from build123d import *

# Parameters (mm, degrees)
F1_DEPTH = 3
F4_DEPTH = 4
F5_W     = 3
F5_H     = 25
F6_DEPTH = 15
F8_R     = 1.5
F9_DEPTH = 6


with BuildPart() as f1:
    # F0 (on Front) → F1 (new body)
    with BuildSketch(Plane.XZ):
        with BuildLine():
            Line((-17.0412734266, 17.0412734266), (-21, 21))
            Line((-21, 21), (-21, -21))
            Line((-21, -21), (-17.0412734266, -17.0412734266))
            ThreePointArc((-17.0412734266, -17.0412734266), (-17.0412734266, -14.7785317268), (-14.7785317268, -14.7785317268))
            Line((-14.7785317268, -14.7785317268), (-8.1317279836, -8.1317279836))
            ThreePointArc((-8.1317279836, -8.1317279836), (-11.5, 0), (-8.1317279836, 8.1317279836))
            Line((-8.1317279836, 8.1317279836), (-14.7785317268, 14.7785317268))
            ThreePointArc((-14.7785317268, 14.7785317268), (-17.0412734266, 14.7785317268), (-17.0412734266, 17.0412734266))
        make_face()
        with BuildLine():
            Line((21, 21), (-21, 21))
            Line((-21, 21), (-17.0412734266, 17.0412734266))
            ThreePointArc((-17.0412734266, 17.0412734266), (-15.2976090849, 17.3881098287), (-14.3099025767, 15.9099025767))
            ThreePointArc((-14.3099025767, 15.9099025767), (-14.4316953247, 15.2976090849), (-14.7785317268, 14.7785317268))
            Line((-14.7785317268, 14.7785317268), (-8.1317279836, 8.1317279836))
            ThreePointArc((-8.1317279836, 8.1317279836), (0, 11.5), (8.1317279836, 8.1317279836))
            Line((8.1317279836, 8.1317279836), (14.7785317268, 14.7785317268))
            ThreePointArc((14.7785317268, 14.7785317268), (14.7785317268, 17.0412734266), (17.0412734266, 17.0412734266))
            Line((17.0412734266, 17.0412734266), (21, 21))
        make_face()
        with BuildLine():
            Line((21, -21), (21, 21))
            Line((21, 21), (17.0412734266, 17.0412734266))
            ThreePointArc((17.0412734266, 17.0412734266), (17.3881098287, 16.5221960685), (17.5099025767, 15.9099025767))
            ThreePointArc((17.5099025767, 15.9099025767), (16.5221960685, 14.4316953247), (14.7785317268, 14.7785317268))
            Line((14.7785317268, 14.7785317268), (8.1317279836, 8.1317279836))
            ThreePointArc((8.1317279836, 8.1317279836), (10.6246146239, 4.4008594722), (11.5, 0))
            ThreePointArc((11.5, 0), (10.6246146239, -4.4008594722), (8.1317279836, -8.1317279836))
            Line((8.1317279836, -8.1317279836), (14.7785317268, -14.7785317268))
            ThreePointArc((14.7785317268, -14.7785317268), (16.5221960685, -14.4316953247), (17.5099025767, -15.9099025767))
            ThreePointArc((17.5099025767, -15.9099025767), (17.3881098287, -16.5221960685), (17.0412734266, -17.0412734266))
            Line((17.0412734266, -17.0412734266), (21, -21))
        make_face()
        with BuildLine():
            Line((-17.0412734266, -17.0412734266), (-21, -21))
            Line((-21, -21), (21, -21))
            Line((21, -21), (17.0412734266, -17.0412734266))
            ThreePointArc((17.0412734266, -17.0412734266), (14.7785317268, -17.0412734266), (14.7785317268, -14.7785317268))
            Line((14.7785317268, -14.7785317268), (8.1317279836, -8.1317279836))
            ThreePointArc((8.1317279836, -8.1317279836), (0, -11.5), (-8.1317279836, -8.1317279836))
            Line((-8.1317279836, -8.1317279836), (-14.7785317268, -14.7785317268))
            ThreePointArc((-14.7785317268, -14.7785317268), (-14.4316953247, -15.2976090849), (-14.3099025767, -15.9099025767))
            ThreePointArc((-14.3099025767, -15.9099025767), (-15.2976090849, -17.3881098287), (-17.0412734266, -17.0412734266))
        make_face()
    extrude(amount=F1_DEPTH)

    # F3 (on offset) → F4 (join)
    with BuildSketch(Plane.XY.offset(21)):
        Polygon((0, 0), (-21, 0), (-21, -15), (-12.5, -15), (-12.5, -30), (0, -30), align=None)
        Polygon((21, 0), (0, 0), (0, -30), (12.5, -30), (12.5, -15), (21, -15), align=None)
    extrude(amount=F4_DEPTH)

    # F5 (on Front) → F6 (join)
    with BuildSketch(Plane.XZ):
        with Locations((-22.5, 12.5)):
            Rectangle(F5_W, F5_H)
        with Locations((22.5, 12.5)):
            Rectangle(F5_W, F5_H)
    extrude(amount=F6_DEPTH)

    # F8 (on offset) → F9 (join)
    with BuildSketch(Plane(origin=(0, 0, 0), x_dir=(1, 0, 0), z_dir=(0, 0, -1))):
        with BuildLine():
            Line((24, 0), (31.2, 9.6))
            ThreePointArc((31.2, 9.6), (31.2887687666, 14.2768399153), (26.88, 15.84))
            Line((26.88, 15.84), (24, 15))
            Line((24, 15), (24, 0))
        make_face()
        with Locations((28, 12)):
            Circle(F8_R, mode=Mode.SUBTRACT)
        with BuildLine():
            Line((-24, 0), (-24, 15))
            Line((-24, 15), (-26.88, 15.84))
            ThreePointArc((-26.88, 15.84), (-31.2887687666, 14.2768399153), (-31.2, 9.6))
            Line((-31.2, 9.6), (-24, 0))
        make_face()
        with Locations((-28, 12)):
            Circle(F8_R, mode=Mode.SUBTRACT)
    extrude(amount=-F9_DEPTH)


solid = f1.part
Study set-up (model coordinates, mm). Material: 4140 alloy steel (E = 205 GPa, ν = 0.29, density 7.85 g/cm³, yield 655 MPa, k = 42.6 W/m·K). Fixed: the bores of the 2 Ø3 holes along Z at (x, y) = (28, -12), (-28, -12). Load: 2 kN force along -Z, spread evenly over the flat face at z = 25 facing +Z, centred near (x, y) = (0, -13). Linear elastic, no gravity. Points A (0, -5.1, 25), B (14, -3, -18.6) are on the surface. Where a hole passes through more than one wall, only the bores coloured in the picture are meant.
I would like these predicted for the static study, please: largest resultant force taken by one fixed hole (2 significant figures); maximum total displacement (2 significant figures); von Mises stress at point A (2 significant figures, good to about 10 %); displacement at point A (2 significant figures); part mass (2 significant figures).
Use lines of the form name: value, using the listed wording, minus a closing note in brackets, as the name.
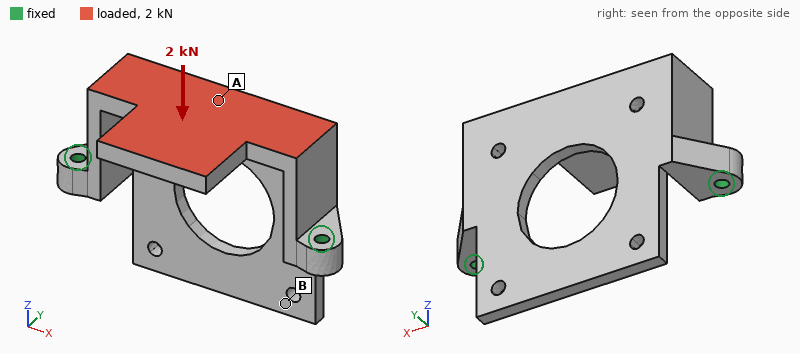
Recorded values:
largest resultant force taken by one fixed hole: 1.0 kN
maximum total displacement: 0.14 mm
von Mises stress at point A: 66 MPa
displacement at point A: 0.023 mm
part mass: 87 g
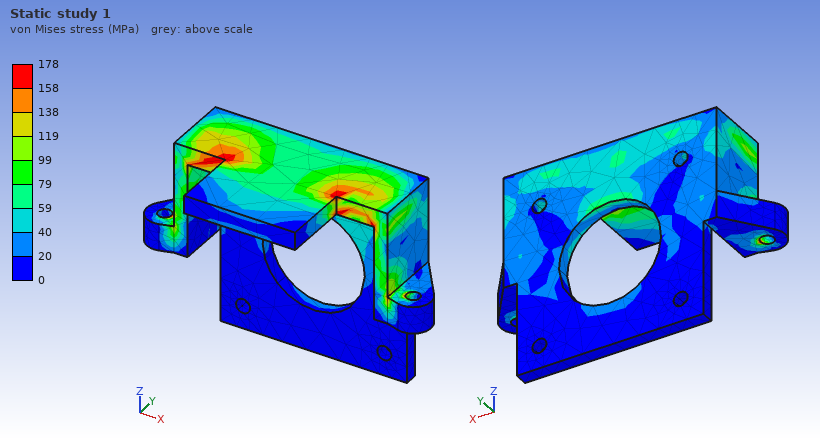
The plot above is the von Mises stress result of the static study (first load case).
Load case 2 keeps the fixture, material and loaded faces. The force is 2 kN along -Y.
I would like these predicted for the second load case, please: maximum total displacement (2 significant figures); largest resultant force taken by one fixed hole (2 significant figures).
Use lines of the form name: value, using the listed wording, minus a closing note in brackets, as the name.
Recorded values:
maximum total displacement: 0.15 mm
largest resultant force taken by one fixed hole: 1.0 kN
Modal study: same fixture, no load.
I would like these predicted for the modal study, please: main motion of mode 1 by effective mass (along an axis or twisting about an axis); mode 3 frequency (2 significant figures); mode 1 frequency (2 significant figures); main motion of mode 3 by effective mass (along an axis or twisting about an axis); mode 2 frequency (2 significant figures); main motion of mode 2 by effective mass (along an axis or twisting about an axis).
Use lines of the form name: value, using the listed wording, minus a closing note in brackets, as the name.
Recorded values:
main motion of mode 1 by effective mass: twisting about X
mode 3 frequency: 4600 Hz
mode 1 frequency: 2400 Hz
main motion of mode 3 by effective mass: along X
mode 2 frequency: 3500 Hz
main motion of mode 2 by effective mass: along Y
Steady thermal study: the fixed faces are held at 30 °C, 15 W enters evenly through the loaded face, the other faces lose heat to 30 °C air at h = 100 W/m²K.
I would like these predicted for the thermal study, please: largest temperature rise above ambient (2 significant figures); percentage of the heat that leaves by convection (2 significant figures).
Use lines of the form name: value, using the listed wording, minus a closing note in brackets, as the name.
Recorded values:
largest temperature rise above ambient: 42 K
percentage of the heat that leaves by convection: 69 %
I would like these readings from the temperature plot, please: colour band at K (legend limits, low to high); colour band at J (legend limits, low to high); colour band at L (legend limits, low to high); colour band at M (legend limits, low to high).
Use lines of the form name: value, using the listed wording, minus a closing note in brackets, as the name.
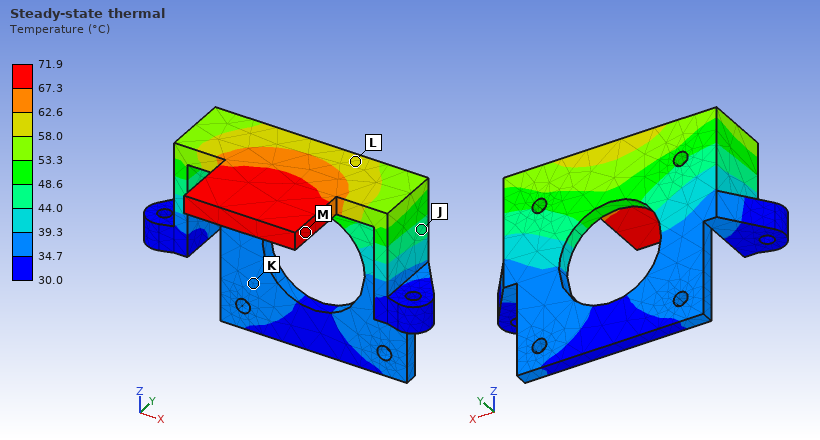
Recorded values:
colour band at K: 34.7 to 39.3 °C
colour band at J: 44.0 to 48.6 °C
colour band at L: 58.0 to 62.6 °C
colour band at M: 67.3 to 71.9 °C
